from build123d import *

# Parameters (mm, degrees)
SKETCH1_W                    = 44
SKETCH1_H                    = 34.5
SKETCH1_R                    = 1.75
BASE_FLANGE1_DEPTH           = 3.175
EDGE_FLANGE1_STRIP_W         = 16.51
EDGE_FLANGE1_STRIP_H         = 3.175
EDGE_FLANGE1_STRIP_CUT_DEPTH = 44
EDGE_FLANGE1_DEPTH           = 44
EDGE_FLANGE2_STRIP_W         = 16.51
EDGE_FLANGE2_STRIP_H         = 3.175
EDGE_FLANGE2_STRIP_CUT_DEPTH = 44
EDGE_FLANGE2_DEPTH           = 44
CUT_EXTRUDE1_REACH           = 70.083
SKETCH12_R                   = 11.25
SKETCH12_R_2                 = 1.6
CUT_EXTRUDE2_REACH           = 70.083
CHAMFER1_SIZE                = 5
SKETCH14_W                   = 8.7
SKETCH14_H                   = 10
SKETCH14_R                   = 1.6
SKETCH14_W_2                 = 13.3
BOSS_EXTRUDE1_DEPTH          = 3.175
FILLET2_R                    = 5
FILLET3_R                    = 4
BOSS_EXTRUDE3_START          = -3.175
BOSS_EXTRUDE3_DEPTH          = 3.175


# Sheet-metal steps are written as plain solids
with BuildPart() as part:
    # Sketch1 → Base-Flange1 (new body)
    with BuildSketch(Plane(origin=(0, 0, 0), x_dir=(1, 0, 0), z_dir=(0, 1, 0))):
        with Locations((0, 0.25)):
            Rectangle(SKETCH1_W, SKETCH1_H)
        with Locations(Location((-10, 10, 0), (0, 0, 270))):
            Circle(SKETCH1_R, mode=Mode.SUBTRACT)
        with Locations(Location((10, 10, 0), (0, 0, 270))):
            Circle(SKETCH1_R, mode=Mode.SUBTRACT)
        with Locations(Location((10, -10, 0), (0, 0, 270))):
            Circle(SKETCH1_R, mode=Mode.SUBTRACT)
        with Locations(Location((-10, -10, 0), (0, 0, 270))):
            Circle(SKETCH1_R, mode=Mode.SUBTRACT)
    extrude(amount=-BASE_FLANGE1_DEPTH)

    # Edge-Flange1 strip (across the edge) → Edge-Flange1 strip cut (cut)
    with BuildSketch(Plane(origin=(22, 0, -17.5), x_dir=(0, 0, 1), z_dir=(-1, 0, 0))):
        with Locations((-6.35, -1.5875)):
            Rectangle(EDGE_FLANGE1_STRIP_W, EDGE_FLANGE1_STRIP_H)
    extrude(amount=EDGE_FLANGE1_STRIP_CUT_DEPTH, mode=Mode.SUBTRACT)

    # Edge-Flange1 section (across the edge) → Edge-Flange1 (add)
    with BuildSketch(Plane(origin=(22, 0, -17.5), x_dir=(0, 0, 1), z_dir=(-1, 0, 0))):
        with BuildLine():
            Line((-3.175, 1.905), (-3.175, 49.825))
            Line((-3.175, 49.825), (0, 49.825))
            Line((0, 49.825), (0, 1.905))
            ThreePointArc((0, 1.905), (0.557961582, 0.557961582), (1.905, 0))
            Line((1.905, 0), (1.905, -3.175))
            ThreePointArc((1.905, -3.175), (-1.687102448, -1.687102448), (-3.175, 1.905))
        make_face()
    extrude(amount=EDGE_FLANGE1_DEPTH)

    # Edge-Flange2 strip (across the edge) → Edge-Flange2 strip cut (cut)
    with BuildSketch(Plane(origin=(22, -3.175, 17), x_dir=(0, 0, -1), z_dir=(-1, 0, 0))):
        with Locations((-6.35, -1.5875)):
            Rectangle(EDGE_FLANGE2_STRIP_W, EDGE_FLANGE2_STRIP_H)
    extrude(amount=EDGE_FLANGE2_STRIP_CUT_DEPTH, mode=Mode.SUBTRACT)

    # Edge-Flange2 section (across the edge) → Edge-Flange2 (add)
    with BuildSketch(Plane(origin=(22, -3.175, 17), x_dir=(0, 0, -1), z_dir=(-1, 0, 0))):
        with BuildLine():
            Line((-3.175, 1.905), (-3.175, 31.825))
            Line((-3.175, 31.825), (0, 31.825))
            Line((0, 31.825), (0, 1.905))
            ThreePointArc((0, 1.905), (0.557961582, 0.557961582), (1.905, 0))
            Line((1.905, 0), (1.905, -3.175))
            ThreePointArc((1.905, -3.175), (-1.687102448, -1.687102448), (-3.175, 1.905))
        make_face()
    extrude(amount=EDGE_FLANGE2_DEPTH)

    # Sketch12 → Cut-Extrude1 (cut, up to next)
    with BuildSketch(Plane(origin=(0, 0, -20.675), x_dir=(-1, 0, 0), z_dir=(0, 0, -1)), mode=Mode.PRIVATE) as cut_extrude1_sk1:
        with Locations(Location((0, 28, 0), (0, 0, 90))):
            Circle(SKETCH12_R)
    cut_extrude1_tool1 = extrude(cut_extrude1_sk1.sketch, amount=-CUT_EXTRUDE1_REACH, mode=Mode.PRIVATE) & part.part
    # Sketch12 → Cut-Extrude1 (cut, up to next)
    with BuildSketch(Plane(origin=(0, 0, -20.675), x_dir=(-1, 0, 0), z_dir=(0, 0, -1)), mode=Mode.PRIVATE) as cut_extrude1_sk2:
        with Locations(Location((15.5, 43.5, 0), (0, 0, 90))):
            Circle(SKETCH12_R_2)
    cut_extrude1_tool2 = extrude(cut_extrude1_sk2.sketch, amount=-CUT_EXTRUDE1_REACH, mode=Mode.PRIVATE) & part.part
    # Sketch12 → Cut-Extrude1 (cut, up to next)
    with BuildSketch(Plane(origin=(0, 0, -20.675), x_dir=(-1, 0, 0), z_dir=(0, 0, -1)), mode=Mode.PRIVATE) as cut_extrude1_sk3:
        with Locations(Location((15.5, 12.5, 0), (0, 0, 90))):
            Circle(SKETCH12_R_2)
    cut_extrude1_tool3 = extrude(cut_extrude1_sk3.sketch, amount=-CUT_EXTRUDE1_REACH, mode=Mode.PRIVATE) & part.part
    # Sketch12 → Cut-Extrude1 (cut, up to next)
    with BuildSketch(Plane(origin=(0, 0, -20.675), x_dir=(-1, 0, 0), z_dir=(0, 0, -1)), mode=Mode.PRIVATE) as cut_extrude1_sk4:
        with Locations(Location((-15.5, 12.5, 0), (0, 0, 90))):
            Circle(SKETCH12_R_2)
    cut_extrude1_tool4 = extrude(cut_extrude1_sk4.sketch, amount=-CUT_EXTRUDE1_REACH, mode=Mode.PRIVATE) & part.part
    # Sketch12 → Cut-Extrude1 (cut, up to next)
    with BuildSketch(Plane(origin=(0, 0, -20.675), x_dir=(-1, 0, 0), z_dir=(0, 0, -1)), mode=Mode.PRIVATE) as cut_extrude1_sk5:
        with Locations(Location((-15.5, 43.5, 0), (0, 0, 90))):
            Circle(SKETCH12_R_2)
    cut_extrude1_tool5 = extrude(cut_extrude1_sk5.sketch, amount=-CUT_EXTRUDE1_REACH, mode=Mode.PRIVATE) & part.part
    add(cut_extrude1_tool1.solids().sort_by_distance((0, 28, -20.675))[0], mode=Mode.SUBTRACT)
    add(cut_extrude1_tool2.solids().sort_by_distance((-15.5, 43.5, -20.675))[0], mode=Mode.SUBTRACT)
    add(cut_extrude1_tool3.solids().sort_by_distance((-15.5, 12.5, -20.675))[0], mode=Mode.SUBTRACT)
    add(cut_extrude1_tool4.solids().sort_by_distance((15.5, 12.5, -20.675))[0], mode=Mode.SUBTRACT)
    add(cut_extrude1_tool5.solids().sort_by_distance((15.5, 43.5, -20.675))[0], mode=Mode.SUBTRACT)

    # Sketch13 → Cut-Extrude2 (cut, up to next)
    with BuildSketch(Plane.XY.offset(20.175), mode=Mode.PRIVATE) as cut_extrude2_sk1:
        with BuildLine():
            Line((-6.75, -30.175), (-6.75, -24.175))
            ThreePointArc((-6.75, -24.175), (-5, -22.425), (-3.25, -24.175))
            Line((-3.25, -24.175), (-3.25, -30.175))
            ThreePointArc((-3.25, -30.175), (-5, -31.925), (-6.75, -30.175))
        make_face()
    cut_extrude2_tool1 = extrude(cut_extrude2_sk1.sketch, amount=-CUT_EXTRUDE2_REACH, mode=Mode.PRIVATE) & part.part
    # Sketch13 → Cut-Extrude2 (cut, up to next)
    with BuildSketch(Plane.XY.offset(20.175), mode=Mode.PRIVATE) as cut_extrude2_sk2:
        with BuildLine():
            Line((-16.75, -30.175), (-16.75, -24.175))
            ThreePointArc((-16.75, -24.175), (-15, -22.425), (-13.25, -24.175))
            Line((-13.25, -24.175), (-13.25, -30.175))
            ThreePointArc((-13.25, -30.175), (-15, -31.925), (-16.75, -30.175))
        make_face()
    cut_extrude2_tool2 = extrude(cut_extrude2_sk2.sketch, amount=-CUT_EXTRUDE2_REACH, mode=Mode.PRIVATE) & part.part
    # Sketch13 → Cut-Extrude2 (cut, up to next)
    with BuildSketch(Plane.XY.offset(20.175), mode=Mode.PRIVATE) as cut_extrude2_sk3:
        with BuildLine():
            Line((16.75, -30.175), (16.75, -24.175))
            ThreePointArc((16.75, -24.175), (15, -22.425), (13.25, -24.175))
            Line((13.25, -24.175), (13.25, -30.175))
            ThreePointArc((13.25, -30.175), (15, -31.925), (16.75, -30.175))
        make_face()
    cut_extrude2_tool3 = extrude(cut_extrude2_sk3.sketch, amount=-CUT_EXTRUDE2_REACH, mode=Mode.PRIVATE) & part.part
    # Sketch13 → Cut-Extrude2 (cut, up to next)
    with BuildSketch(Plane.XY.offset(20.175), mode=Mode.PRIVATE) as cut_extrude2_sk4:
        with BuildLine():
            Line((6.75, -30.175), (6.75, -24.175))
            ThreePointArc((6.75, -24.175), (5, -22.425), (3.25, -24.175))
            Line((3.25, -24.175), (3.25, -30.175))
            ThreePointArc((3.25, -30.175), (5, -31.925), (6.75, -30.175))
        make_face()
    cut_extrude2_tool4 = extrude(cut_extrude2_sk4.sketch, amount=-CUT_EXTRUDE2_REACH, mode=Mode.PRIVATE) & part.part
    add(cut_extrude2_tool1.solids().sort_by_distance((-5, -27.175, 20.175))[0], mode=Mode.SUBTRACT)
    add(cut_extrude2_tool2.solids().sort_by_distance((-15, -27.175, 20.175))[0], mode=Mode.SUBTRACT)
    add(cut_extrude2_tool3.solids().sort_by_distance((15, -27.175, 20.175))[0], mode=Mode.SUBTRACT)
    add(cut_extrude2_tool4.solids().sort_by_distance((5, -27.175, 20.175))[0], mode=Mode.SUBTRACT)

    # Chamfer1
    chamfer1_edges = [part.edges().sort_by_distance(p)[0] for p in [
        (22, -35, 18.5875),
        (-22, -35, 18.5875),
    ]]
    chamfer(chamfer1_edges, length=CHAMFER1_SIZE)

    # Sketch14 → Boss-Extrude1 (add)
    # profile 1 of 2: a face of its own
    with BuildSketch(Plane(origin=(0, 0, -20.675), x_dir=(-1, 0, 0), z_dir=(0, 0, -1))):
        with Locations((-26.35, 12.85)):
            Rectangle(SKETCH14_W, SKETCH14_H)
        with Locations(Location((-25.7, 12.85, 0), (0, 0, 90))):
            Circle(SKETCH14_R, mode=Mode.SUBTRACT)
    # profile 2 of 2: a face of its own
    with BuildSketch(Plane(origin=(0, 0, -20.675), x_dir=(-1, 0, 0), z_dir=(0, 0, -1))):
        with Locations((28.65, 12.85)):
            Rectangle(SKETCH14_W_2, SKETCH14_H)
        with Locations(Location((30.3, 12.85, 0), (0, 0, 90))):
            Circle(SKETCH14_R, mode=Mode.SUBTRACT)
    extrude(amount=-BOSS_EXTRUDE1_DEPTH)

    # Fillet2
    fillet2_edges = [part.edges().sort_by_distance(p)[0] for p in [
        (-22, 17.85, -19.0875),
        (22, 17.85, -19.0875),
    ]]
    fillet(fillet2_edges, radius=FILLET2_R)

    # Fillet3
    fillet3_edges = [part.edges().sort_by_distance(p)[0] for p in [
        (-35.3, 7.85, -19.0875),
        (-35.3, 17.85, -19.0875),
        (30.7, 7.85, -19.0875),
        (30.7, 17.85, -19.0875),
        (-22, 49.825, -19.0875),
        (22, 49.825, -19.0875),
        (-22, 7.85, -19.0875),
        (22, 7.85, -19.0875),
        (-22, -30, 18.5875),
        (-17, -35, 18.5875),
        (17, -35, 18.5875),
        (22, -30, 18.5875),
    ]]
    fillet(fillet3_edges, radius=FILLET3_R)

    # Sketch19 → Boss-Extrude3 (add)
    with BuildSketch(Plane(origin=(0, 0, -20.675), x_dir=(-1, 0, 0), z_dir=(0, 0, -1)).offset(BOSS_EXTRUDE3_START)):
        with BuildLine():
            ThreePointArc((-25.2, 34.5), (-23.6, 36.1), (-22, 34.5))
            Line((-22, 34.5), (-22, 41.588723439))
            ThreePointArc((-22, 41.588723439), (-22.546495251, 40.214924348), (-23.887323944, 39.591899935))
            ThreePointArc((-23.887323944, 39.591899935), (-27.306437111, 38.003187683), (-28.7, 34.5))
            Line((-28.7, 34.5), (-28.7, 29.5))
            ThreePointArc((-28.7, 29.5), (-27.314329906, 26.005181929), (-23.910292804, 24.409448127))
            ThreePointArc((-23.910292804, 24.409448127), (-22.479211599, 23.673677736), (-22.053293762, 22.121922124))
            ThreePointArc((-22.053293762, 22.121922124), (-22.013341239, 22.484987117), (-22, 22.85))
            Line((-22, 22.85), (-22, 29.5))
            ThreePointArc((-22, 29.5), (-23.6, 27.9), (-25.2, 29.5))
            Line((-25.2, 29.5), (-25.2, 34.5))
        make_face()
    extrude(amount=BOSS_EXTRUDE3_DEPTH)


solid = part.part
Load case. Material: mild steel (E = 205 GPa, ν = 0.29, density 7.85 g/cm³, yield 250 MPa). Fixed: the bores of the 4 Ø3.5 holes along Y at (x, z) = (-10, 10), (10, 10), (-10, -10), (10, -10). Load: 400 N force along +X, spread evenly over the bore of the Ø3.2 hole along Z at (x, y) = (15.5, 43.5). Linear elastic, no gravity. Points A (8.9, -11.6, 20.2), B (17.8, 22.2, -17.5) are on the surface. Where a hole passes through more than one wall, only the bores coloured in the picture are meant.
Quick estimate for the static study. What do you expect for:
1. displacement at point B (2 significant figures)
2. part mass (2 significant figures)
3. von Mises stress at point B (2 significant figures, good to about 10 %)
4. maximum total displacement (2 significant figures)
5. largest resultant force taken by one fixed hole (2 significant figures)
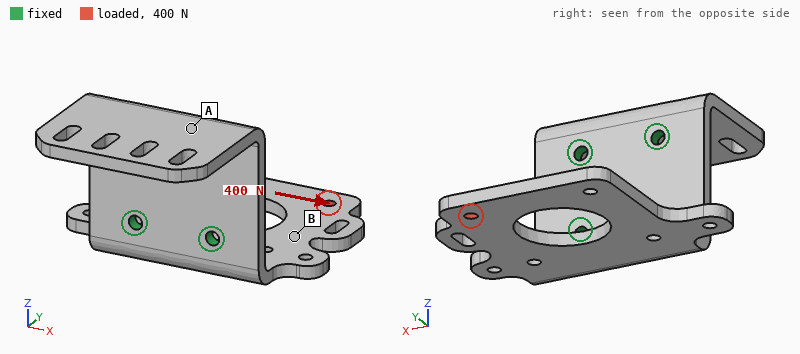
39 µm
120 g
22 MPa
72 µm
830 N
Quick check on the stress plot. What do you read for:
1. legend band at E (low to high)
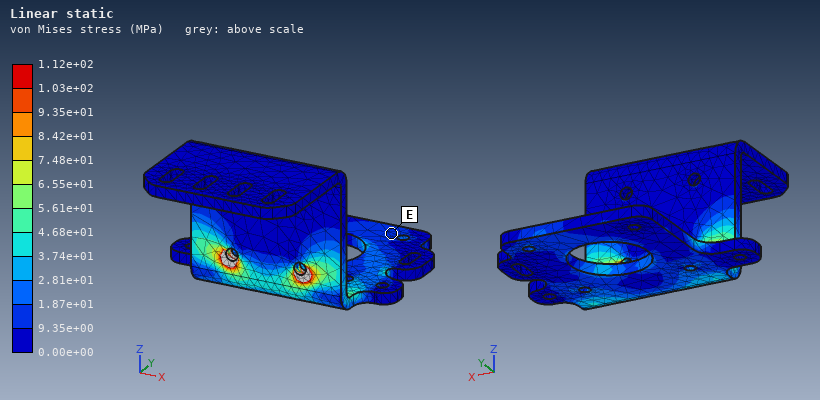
9.35e+00 to 1.87e+01 MPa
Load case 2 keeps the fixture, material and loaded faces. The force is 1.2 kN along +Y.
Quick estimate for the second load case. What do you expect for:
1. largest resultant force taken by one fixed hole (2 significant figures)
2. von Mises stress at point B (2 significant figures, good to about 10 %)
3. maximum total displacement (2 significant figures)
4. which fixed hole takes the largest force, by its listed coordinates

1.5 kN
34 MPa
0.16 mm
(10, -10)
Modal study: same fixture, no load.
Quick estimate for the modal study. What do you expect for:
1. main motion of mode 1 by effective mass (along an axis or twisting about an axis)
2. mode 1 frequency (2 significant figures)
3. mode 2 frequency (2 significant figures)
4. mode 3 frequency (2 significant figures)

along Z
820 Hz
1900 Hz
2000 Hz
